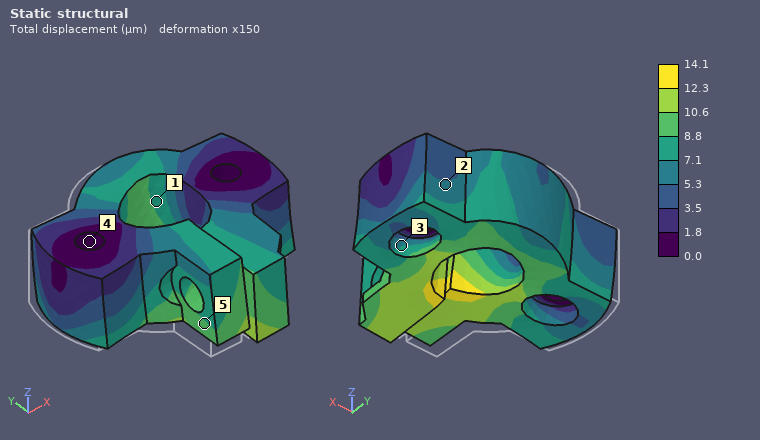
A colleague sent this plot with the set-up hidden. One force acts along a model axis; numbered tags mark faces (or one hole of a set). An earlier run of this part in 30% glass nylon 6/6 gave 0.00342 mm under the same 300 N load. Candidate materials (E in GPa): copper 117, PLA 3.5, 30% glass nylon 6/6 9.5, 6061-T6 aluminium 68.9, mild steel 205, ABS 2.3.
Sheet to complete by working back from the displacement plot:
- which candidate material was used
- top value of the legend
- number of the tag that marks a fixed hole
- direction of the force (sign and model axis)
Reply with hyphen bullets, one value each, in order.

- ABS
- 14.1 µm
- 4
- +X
